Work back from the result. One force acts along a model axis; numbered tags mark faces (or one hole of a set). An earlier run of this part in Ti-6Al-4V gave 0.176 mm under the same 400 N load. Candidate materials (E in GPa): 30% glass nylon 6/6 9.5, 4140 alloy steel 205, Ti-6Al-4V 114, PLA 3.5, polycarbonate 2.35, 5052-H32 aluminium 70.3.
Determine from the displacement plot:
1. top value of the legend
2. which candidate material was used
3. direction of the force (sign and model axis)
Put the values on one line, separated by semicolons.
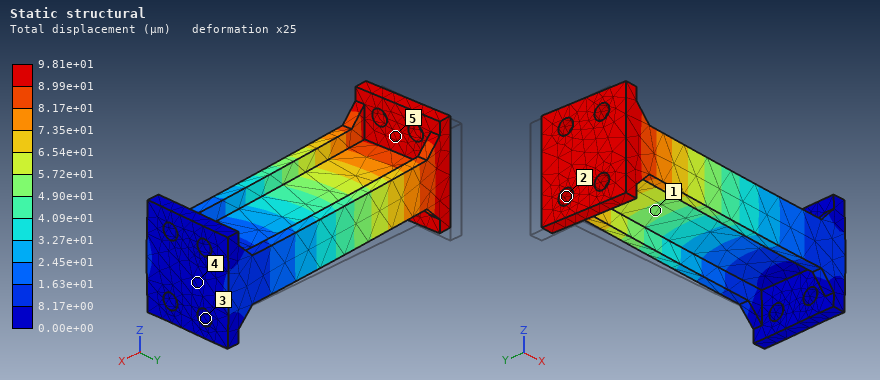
9.81e+01 µm; 4140 alloy steel; -Y
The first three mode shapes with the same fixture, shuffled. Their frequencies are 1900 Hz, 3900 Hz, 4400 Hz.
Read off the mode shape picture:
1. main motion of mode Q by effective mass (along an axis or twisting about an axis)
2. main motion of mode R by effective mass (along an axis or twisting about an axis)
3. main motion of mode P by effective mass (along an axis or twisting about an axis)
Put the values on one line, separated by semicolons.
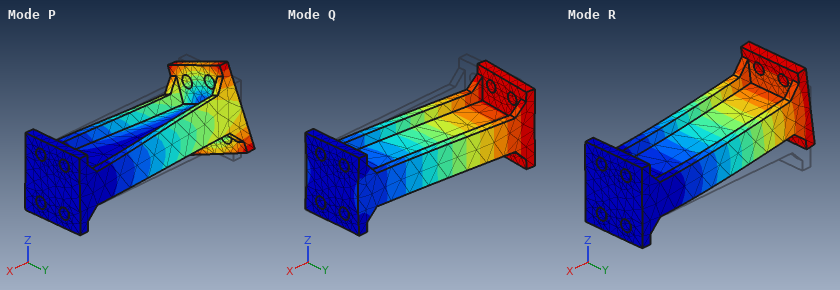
along Y; along Z; twisting about X
